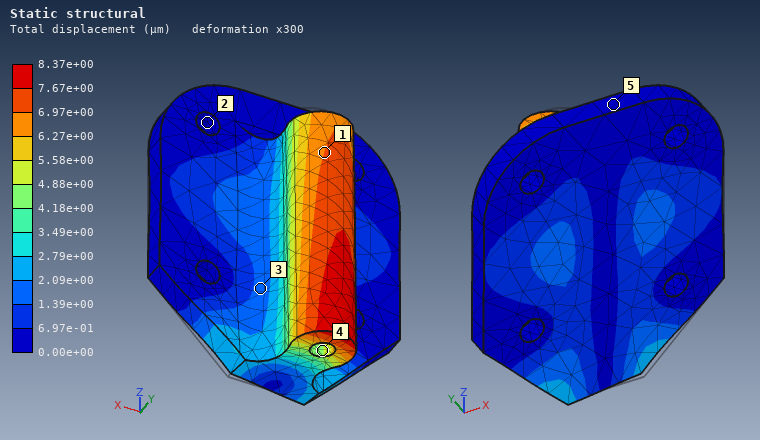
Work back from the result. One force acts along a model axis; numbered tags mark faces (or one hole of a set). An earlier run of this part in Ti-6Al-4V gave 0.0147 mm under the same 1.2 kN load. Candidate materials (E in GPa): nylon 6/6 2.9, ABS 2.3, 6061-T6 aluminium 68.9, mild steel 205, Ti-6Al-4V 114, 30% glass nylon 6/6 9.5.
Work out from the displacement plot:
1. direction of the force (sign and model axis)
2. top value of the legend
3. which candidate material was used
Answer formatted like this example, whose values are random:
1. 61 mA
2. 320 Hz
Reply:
1. -X
2. 8.37e+00 µm
3. mild steel
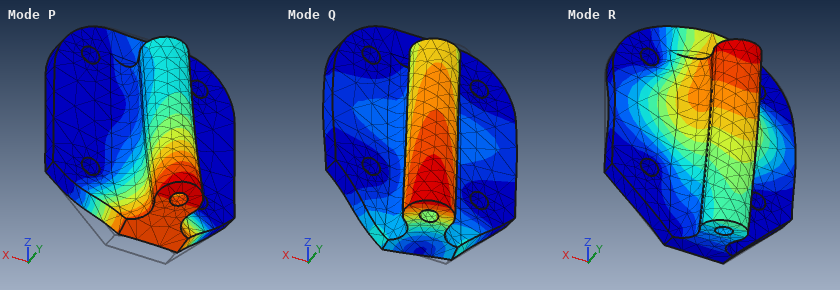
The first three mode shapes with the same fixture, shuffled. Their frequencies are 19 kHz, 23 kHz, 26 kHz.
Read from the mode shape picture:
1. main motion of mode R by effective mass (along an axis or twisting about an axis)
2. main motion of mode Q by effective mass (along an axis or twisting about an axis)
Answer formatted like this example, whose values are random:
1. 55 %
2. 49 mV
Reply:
1. along Y
2. along X
